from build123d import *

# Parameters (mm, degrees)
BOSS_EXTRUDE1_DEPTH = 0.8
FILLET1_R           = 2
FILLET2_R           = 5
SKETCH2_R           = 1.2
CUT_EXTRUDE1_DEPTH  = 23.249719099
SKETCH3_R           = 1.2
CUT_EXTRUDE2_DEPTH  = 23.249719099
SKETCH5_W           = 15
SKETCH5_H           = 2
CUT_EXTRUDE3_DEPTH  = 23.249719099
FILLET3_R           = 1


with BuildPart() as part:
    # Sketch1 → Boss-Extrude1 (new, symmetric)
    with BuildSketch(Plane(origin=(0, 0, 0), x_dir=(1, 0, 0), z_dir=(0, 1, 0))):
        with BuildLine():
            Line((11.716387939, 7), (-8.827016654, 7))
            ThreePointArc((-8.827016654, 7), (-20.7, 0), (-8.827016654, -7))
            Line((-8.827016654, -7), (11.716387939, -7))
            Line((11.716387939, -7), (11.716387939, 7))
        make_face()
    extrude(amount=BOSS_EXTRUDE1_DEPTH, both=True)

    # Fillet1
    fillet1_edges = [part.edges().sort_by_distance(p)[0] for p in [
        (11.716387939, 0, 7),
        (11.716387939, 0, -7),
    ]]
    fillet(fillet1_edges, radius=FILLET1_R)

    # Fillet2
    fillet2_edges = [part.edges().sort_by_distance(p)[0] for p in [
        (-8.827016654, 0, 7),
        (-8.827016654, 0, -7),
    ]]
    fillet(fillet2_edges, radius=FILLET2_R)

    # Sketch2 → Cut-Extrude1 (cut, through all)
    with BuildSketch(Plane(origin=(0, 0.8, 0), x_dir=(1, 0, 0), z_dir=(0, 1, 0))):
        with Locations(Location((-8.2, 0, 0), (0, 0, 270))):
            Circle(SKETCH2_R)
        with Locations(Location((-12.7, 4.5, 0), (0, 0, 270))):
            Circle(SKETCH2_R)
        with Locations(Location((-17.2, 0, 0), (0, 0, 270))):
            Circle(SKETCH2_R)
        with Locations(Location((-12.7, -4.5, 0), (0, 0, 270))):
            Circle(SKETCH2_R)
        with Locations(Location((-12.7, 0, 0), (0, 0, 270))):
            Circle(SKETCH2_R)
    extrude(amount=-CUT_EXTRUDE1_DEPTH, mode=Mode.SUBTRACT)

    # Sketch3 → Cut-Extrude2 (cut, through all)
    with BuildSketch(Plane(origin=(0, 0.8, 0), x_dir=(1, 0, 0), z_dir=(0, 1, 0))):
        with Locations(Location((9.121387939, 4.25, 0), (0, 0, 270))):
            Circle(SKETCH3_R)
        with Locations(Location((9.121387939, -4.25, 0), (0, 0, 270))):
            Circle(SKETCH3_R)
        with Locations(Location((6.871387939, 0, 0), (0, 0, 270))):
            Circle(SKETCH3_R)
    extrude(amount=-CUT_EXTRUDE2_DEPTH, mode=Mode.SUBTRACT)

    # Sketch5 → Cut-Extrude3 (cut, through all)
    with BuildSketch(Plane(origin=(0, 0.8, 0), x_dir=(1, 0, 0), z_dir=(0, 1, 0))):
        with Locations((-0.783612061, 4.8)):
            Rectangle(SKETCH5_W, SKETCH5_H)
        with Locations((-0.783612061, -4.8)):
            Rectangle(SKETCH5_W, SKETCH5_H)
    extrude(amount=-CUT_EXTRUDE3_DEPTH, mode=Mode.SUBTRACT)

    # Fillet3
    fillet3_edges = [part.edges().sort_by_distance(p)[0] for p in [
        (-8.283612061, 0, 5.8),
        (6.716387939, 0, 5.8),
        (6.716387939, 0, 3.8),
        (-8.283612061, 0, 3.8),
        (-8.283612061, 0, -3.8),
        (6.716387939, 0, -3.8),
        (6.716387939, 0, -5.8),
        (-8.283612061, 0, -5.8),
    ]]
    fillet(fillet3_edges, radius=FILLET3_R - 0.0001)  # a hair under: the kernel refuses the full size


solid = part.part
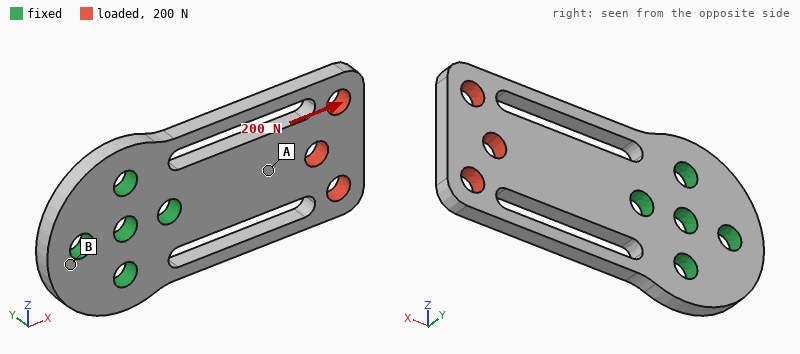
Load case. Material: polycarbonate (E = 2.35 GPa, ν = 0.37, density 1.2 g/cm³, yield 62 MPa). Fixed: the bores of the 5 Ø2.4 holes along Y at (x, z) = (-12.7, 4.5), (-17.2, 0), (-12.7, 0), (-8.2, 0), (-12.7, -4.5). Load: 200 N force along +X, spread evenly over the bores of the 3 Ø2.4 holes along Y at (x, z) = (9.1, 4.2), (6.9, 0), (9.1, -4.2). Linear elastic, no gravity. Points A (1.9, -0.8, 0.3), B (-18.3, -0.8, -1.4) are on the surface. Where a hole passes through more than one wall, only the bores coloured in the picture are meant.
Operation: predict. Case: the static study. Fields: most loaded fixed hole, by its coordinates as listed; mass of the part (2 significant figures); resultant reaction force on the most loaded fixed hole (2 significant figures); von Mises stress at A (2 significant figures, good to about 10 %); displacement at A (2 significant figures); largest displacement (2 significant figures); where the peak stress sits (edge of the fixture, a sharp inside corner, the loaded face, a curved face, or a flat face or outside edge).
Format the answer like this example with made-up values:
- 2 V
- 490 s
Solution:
- (-8.2, 0)
- 0.68 g
- 120 N
- 12 MPa
- 0.056 mm
- 0.11 mm
- the loaded face
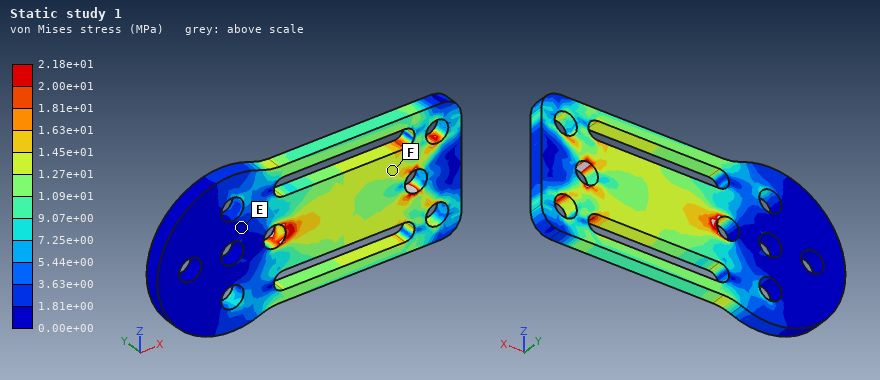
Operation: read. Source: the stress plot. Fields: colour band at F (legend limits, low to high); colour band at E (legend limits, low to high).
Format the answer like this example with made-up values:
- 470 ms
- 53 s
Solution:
- 1.27e+01 to 1.45e+01 MPa
- 0.00e+00 to 1.81e+00 MPa
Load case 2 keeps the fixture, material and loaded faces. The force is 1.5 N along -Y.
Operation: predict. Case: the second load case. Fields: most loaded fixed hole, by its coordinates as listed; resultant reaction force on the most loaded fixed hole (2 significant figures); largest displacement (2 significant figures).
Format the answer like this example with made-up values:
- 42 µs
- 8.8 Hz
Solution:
- (-8.2, 0)
- 3.2 N
- 0.34 mm
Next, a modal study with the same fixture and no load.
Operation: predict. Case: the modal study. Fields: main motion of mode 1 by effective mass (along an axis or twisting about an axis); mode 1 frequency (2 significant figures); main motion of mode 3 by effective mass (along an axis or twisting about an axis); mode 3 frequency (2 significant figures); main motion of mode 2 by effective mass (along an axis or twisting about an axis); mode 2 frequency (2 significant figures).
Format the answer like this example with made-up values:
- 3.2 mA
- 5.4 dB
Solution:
- along Y
- 910 Hz
- along Z
- 3900 Hz
- twisting about X
- 2400 Hz
